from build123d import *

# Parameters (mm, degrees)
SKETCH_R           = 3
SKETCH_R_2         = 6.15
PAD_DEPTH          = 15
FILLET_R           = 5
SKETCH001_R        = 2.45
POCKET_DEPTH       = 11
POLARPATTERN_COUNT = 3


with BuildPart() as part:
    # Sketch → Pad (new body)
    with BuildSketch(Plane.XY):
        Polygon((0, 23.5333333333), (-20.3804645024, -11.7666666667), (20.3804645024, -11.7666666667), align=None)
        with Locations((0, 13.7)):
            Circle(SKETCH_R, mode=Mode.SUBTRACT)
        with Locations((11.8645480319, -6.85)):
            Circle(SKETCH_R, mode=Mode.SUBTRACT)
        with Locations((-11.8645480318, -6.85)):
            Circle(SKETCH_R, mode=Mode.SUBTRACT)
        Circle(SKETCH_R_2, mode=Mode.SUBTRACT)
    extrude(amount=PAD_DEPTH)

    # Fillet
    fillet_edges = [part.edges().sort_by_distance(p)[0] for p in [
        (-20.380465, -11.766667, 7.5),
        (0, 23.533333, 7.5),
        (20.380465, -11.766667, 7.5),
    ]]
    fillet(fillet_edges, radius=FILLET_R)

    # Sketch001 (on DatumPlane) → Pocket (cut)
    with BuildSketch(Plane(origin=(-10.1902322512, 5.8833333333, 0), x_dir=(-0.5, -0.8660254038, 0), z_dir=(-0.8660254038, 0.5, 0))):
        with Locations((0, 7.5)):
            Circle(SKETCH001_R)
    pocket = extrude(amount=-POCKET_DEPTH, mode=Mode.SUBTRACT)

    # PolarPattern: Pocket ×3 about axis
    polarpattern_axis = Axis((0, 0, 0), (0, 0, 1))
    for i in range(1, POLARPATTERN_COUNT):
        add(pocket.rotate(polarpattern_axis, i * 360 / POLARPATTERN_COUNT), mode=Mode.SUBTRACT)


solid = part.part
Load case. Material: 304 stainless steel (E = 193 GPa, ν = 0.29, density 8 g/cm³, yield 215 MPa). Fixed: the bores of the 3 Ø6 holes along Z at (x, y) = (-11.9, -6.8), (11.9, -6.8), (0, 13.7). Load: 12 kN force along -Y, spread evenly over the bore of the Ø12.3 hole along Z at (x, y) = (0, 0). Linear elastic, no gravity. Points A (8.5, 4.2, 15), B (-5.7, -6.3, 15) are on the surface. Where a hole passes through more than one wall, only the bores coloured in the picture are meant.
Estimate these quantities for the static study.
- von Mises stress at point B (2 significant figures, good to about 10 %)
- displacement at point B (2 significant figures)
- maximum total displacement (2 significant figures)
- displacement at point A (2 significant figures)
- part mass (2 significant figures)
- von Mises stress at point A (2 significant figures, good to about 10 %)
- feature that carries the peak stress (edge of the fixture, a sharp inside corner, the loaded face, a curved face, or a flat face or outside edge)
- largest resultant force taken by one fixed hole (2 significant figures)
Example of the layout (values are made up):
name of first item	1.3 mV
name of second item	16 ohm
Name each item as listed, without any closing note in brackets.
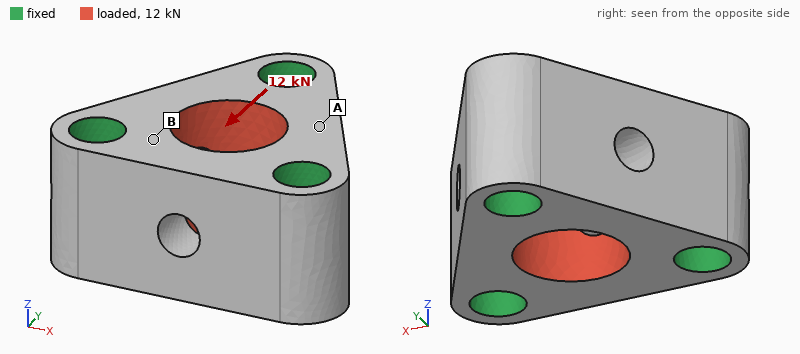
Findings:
von Mises stress at point B	34 MPa
displacement at point B	1.6 µm
maximum total displacement	3.5 µm
displacement at point A	1.7 µm
part mass	53 g
von Mises stress at point A	13 MPa
feature that carries the peak stress	edge of the fixture
largest resultant force taken by one fixed hole	4.1 kN
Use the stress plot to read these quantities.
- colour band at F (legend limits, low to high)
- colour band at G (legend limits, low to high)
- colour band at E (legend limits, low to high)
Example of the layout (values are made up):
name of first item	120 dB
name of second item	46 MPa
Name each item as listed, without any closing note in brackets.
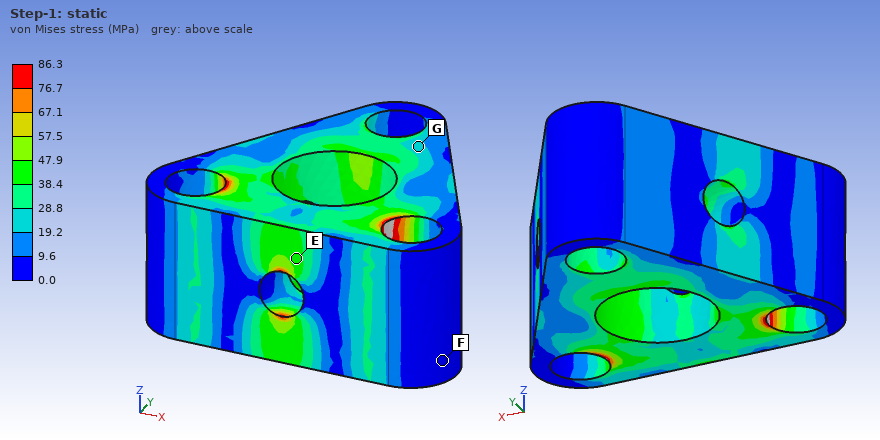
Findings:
colour band at F	0.0 to 9.6 MPa
colour band at G	19.2 to 28.8 MPa
colour band at E	38.4 to 47.9 MPa
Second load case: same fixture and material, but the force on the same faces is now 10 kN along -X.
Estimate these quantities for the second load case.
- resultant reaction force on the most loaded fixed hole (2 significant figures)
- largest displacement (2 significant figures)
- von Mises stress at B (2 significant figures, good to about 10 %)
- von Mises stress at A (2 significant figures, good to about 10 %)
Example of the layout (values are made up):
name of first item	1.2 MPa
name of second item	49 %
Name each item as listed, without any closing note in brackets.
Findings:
resultant reaction force on the most loaded fixed hole	3.4 kN
largest displacement	2.6 µm
von Mises stress at B	27 MPa
von Mises stress at A	16 MPa
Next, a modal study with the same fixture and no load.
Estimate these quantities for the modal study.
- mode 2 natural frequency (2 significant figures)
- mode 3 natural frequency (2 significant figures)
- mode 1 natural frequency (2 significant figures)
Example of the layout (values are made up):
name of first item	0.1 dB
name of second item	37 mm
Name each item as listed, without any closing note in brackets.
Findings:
mode 2 natural frequency	66 kHz
mode 3 natural frequency	74 kHz
mode 1 natural frequency	66 kHz
